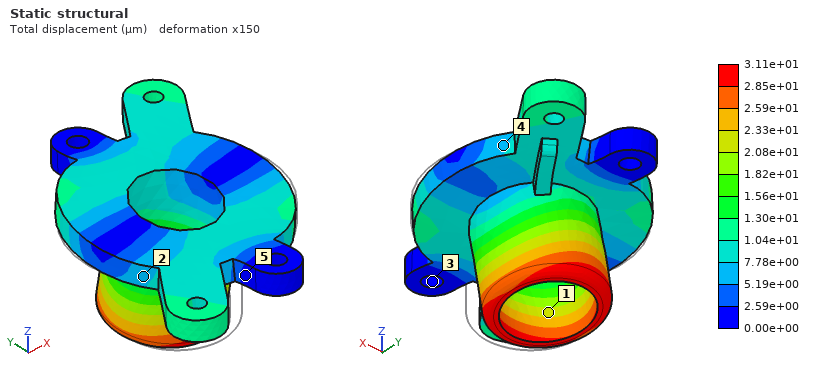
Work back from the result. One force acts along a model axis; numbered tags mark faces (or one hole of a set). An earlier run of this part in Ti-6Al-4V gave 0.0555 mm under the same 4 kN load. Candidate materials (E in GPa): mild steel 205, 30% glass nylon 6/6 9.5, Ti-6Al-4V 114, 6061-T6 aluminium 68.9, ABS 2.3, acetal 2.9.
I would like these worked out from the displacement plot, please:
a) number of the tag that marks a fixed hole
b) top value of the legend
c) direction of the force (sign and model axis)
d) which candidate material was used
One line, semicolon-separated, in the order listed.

3; 3.11e+01 µm; +Y; mild steel
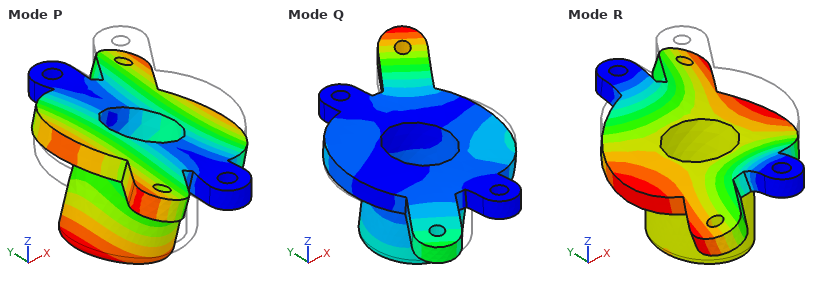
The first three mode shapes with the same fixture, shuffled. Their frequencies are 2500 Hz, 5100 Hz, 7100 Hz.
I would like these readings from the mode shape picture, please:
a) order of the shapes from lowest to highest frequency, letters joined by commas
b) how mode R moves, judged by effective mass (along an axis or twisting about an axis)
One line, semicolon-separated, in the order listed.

P, R, Q; along Z
